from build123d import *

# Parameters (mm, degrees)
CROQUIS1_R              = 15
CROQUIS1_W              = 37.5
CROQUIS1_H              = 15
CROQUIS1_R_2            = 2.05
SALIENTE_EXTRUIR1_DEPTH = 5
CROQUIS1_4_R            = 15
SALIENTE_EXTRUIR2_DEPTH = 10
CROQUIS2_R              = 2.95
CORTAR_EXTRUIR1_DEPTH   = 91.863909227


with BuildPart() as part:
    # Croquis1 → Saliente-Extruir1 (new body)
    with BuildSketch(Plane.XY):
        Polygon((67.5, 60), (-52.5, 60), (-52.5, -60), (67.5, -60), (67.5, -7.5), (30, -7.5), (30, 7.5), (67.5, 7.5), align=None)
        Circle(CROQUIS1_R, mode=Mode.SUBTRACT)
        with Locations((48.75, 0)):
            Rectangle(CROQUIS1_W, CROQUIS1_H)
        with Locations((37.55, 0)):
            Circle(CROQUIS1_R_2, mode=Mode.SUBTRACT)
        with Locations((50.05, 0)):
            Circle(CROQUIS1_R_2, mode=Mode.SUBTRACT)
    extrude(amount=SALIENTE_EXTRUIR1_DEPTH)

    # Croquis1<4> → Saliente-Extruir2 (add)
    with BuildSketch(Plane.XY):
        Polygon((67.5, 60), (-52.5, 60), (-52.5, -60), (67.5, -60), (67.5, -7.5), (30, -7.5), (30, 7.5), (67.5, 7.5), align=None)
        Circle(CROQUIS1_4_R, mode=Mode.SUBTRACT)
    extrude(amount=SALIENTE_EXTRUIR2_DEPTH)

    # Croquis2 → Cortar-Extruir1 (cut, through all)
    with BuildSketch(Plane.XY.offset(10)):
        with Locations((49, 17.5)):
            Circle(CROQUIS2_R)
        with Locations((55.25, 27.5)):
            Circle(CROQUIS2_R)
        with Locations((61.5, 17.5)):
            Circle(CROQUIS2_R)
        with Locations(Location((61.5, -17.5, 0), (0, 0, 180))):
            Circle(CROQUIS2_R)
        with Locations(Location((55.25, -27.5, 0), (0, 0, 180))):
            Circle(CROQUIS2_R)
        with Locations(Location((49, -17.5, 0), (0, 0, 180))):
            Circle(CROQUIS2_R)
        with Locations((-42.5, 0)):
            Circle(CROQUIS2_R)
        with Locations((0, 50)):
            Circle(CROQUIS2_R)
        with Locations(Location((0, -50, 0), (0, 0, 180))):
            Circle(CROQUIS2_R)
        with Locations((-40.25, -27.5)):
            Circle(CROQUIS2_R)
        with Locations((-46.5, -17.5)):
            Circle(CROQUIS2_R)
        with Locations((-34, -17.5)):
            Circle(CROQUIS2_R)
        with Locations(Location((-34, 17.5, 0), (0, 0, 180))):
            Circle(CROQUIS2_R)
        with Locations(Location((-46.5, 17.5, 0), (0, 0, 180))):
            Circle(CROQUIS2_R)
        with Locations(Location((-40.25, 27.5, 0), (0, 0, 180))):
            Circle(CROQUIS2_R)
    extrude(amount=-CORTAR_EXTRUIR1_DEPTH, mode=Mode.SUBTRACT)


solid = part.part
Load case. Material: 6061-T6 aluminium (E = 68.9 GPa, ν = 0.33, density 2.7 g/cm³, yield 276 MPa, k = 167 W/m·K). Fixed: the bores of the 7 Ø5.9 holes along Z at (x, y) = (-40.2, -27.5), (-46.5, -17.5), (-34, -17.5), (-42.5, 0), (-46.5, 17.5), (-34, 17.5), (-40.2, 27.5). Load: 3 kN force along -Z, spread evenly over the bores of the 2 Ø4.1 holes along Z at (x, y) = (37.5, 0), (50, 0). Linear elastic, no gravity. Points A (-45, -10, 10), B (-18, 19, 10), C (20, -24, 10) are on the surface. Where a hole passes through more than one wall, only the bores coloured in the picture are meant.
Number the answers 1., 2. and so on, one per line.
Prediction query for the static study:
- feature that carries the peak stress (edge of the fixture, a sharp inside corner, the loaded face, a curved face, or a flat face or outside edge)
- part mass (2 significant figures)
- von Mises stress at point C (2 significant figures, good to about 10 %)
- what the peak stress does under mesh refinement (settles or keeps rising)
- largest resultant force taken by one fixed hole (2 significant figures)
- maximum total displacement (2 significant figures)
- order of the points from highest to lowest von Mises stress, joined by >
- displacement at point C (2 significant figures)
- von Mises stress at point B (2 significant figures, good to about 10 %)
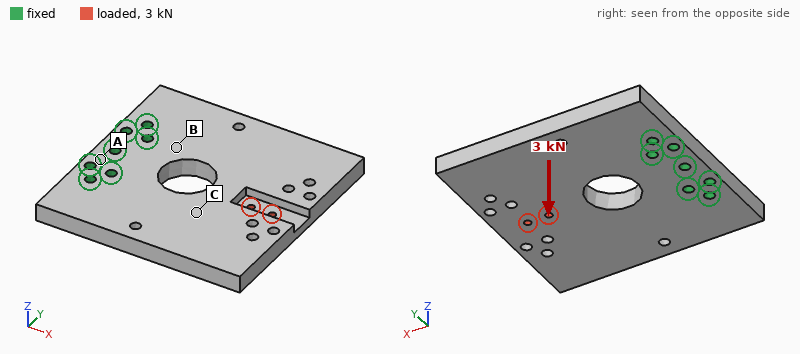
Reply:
1. edge of the fixture
2. 350 g
3. 53 MPa
4. keeps rising
5. 4.0 kN
6. 1.4 mm
7. B > C > A
8. 0.55 mm
9. 120 MPa
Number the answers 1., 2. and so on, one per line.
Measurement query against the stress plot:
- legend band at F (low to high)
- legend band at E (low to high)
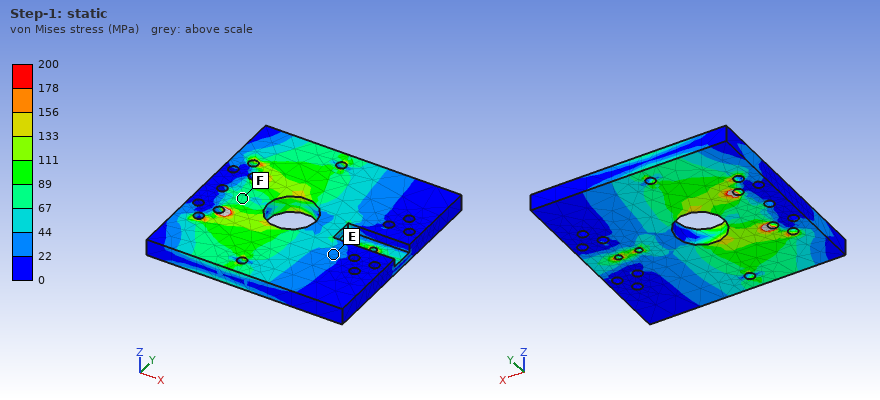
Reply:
1. 67 to 89 MPa
2. 22 to 44 MPa
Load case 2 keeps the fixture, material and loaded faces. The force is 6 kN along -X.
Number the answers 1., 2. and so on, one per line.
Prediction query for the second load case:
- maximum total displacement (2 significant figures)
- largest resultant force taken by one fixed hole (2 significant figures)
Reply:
1. 0.16 mm
2. 1.8 kN
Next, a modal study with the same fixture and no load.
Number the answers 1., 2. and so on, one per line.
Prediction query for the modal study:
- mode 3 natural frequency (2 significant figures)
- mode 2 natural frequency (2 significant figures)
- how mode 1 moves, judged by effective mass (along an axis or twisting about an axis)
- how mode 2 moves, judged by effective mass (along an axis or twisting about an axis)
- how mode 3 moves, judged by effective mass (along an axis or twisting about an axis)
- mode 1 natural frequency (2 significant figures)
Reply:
1. 3200 Hz
2. 1300 Hz
3. along Z
4. twisting about X
5. along Y
6. 710 Hz
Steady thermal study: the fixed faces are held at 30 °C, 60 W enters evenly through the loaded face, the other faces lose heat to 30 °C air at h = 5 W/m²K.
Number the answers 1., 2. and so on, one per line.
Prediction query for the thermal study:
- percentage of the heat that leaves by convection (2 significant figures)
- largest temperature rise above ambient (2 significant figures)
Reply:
1. 4.9 %
2. 47 K
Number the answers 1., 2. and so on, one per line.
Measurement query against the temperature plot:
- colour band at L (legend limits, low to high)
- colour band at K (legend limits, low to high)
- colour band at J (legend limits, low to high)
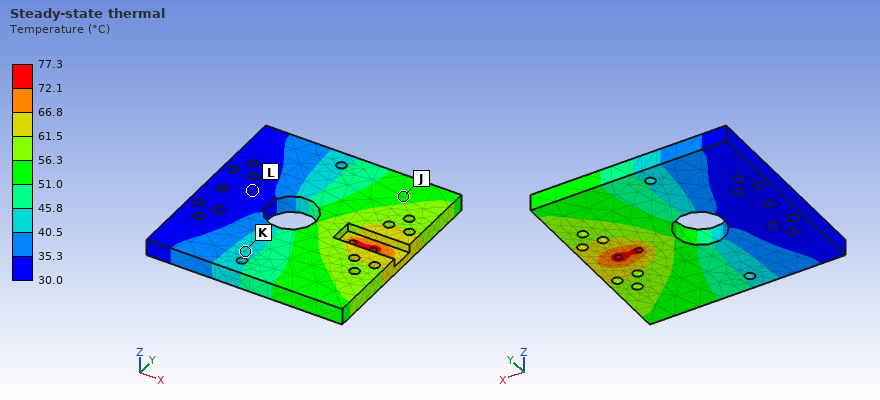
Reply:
1. 30.0 to 35.3 °C
2. 40.5 to 45.8 °C
3. 51.0 to 56.3 °C
